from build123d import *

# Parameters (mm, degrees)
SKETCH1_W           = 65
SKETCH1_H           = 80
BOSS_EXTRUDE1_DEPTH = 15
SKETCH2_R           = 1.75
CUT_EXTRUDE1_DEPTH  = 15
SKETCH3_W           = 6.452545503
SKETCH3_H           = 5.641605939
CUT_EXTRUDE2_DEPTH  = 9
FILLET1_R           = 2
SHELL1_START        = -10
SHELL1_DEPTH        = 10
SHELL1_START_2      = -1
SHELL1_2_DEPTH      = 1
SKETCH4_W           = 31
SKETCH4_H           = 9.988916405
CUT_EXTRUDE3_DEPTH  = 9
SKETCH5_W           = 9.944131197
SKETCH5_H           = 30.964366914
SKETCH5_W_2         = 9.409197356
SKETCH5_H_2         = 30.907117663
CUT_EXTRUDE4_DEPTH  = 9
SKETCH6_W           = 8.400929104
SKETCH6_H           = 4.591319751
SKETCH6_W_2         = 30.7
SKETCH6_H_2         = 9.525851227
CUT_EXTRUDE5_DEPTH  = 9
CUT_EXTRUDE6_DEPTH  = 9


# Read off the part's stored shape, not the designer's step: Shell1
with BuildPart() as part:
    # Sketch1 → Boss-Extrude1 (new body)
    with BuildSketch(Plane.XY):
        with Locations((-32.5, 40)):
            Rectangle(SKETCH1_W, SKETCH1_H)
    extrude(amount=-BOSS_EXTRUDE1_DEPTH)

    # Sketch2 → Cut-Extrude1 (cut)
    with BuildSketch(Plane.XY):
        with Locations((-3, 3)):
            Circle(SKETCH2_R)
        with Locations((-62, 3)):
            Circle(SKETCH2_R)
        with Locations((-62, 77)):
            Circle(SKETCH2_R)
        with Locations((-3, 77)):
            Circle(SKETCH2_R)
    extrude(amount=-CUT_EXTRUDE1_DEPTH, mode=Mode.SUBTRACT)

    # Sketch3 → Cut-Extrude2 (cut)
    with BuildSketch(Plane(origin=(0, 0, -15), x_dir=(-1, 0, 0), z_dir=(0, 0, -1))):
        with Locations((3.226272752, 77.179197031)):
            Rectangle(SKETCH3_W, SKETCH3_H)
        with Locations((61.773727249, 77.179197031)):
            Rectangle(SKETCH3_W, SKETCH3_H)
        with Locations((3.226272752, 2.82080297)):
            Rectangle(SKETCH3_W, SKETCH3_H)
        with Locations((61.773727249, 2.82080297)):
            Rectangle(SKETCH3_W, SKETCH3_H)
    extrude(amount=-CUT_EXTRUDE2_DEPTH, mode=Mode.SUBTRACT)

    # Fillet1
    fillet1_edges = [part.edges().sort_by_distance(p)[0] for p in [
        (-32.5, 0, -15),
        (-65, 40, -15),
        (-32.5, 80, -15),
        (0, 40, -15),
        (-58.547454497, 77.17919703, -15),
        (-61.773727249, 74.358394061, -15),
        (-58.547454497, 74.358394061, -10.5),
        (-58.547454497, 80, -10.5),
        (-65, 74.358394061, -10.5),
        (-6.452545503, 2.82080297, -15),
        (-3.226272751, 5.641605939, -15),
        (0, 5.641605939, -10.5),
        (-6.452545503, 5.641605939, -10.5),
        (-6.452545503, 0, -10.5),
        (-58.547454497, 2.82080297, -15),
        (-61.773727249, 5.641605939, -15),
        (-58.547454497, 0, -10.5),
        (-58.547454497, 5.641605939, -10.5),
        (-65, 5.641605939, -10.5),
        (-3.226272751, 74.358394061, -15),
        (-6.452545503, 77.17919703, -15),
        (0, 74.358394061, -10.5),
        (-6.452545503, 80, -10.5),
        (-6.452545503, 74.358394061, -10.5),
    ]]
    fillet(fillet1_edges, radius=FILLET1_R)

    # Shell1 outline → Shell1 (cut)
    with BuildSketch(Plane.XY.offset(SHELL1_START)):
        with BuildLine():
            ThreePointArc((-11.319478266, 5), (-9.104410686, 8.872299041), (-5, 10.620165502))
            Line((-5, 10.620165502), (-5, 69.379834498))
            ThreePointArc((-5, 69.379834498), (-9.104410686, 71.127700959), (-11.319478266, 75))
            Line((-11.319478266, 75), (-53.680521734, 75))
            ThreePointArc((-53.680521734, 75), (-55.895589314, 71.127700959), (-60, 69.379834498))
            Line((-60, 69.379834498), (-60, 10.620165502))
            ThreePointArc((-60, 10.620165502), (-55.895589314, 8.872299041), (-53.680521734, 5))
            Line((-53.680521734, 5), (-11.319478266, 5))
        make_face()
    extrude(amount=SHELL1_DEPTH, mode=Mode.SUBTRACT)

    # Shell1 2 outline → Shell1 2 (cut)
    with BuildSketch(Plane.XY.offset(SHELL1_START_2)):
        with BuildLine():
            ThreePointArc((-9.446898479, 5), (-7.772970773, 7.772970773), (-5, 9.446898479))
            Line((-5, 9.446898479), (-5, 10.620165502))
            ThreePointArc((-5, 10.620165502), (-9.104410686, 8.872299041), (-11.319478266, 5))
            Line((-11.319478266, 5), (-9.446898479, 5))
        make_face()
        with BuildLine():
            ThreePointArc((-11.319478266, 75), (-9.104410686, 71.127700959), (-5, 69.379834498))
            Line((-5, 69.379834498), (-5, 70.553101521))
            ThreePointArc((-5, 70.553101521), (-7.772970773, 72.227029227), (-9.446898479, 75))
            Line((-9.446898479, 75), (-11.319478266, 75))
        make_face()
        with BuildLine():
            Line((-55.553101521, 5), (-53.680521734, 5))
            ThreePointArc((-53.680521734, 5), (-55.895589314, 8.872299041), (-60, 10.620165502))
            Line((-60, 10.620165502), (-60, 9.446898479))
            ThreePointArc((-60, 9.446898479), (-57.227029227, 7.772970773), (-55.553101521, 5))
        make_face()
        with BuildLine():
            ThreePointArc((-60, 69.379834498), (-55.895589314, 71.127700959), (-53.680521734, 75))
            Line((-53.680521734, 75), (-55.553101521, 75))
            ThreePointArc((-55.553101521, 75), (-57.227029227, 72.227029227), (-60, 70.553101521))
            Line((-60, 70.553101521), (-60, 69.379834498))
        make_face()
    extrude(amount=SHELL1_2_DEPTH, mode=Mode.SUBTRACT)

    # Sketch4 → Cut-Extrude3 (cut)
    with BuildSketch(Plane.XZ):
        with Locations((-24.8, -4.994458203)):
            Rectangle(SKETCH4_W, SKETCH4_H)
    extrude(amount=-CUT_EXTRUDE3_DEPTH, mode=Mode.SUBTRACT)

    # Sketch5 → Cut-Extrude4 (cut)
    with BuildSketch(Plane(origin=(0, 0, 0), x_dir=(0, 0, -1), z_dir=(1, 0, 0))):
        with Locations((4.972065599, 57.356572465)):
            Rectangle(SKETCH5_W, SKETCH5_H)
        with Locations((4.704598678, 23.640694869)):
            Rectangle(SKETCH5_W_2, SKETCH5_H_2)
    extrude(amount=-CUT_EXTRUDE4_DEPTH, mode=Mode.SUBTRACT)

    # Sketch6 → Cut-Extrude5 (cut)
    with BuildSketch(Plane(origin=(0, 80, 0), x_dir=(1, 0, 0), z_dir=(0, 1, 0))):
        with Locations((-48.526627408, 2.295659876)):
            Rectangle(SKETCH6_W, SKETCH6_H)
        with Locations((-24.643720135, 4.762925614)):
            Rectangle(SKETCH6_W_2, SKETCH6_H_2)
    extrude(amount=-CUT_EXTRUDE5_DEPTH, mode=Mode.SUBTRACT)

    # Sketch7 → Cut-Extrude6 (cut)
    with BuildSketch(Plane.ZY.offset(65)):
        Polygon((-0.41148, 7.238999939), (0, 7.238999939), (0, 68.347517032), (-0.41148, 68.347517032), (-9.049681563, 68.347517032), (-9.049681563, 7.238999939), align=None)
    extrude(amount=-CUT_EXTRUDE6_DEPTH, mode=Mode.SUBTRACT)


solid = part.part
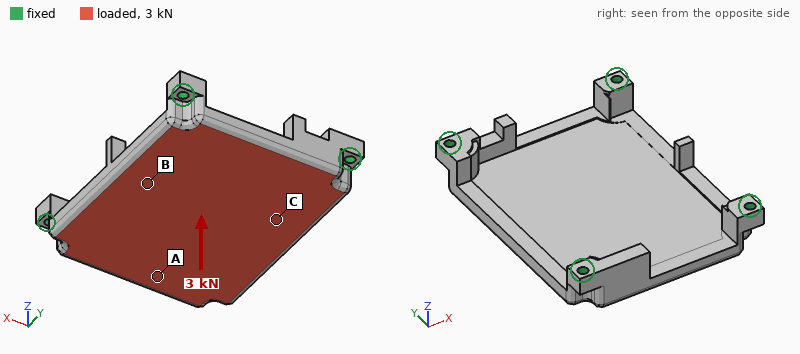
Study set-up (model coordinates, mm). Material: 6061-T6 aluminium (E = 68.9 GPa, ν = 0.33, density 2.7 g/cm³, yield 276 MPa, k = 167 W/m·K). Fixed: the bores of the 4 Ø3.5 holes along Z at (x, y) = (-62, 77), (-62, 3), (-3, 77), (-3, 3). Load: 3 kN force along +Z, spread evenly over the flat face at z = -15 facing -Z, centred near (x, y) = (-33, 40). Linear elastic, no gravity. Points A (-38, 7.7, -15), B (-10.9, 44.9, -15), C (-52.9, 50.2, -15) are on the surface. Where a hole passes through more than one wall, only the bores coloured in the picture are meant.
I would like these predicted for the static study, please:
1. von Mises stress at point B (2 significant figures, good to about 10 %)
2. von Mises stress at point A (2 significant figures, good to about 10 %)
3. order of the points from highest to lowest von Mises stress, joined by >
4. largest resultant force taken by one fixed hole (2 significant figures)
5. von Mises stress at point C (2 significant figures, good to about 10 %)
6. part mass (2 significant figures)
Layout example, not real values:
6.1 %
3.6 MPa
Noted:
44 MPa
23 MPa
B > C > A
1.4 kN
33 MPa
79 g
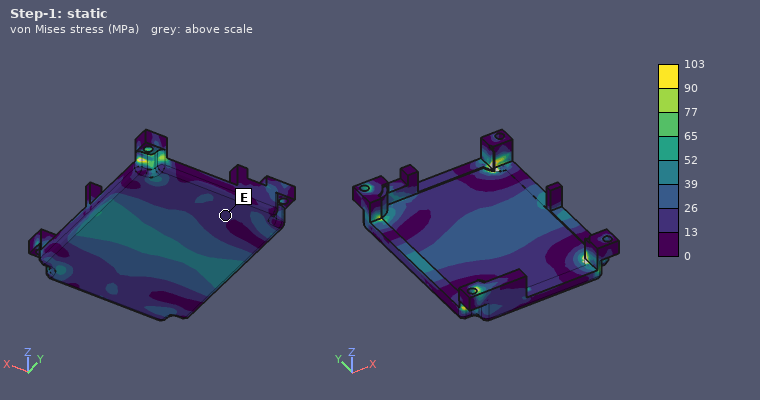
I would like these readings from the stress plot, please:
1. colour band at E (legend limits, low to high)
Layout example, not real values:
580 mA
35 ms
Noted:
13 to 26 MPa
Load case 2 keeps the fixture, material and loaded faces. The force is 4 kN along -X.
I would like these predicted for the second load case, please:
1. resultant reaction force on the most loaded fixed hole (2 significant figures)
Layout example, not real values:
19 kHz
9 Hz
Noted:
1.3 kN
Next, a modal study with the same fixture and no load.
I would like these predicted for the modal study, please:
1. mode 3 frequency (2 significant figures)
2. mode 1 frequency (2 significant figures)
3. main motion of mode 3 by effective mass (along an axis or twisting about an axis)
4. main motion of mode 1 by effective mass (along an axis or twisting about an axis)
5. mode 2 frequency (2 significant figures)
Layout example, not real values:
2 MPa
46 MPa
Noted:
6400 Hz
3800 Hz
along Y
along Z
5600 Hz
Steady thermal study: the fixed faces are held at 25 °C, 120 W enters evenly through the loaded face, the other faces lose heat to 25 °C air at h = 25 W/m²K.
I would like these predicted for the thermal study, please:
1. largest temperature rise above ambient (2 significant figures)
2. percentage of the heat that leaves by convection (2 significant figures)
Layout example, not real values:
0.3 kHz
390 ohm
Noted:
53 K
7.1 %
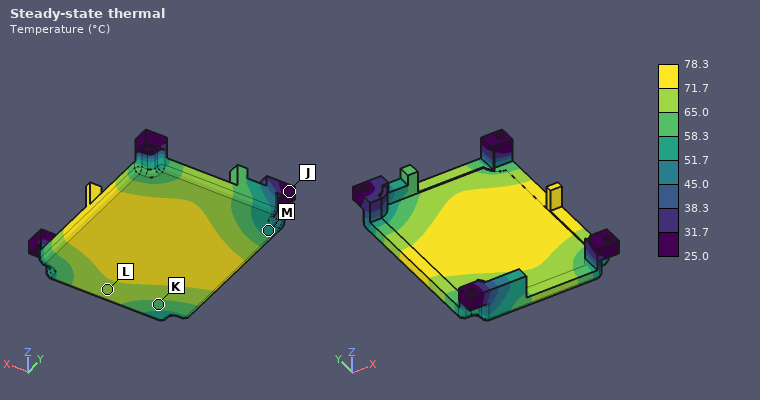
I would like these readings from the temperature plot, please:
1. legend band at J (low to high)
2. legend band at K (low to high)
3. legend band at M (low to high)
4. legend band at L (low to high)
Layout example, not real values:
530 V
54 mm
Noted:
25.0 to 31.7 °C
58.3 to 65.0 °C
51.7 to 58.3 °C
65.0 to 71.7 °C
